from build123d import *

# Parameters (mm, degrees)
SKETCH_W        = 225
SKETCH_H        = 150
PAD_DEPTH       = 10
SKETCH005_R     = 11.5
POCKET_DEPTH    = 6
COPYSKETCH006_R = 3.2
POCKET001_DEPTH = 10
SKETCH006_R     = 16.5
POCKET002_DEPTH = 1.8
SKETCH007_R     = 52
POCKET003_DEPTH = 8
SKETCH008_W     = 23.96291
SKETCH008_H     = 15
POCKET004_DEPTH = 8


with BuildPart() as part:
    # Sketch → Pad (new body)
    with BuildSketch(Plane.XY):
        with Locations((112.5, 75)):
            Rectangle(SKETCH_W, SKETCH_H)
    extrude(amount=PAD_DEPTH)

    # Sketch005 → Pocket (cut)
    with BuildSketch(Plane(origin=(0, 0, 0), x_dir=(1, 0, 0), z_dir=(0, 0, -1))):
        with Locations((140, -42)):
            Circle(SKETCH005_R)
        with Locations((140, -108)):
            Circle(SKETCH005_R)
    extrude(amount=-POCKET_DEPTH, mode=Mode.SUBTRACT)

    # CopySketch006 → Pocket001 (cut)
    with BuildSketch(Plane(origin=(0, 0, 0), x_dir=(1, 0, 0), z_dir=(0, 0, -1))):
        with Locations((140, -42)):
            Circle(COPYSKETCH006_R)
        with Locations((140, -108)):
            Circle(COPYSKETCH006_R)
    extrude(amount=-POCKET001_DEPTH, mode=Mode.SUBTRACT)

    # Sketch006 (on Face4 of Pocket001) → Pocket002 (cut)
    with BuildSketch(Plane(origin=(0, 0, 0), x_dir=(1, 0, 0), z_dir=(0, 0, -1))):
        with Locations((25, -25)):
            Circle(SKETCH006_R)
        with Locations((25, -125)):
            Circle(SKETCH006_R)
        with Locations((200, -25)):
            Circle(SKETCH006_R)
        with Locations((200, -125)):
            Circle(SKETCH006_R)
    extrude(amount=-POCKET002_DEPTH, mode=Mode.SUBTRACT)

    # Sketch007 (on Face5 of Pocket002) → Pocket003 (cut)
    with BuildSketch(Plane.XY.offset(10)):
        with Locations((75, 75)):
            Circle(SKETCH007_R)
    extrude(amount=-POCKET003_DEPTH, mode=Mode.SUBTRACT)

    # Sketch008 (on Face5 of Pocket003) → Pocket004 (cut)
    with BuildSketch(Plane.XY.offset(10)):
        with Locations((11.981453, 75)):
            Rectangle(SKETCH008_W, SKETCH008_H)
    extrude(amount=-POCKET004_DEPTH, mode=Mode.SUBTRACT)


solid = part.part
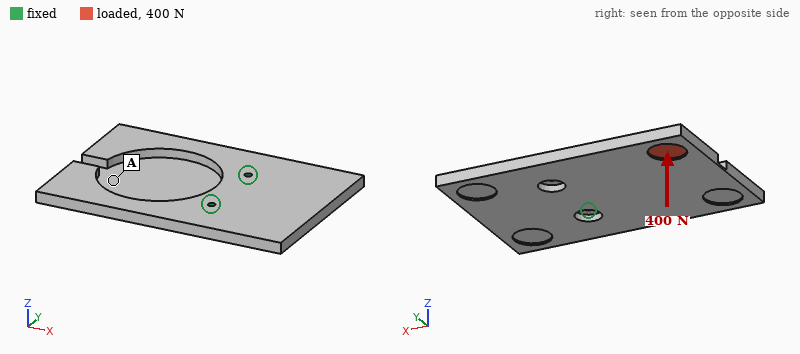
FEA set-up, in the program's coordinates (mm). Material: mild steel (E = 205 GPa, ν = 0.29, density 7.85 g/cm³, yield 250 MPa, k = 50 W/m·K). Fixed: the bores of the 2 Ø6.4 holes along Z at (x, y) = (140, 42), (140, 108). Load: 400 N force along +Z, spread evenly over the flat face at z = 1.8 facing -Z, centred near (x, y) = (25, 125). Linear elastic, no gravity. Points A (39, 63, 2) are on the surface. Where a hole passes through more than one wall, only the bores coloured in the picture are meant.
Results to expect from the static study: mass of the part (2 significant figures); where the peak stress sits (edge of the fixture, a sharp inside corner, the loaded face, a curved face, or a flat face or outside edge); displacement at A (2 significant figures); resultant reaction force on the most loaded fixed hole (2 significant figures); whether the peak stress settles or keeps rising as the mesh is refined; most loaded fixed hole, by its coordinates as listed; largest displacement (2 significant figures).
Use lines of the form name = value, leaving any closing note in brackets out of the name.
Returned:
mass of the part = 2.0 kg
where the peak stress sits = edge of the fixture
displacement at A = 0.27 mm
resultant reaction force on the most loaded fixed hole = 550 N
whether the peak stress settles or keeps rising as the mesh is refined = keeps rising
most loaded fixed hole, by its coordinates as listed = (140, 108)
largest displacement = 0.51 mm
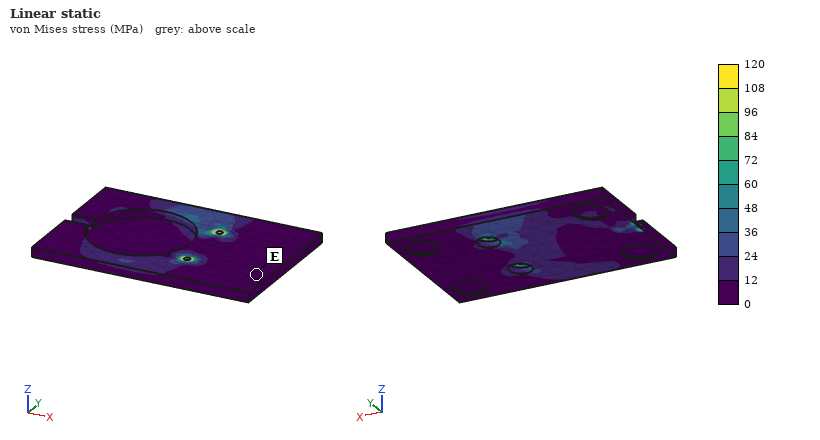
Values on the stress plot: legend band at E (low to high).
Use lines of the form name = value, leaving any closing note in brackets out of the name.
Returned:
legend band at E = 0 to 12 MPa
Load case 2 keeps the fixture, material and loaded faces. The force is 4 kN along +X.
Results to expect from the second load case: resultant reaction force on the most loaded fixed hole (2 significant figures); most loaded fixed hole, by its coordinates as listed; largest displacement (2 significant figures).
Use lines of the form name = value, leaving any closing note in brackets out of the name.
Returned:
resultant reaction force on the most loaded fixed hole = 4.9 kN
most loaded fixed hole, by its coordinates as listed = (140, 108)
largest displacement = 0.23 mm
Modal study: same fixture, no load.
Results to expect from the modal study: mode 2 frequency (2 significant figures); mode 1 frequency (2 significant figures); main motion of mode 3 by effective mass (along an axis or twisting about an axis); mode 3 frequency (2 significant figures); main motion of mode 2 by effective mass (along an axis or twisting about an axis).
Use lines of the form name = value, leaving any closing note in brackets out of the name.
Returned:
mode 2 frequency = 600 Hz
mode 1 frequency = 220 Hz
main motion of mode 3 by effective mass = along Z
mode 3 frequency = 690 Hz
main motion of mode 2 by effective mass = twisting about X
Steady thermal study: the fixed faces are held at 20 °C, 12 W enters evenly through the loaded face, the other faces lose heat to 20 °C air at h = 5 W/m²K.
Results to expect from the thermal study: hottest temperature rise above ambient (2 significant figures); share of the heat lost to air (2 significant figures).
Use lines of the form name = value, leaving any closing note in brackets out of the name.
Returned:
hottest temperature rise above ambient = 45 K
share of the heat lost to air = 41 %
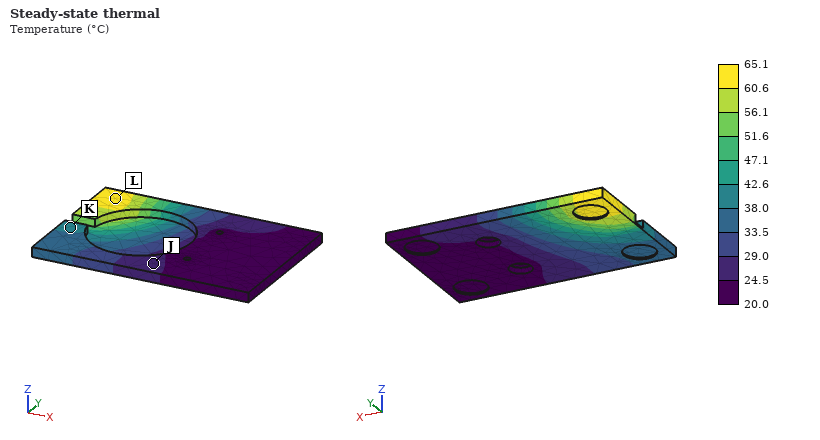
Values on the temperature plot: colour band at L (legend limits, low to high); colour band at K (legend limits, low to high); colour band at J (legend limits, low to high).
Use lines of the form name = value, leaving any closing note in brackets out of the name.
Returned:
colour band at L = 60.6 to 65.1 °C
colour band at K = 38.0 to 42.6 °C
colour band at J = 24.5 to 29.0 °C
